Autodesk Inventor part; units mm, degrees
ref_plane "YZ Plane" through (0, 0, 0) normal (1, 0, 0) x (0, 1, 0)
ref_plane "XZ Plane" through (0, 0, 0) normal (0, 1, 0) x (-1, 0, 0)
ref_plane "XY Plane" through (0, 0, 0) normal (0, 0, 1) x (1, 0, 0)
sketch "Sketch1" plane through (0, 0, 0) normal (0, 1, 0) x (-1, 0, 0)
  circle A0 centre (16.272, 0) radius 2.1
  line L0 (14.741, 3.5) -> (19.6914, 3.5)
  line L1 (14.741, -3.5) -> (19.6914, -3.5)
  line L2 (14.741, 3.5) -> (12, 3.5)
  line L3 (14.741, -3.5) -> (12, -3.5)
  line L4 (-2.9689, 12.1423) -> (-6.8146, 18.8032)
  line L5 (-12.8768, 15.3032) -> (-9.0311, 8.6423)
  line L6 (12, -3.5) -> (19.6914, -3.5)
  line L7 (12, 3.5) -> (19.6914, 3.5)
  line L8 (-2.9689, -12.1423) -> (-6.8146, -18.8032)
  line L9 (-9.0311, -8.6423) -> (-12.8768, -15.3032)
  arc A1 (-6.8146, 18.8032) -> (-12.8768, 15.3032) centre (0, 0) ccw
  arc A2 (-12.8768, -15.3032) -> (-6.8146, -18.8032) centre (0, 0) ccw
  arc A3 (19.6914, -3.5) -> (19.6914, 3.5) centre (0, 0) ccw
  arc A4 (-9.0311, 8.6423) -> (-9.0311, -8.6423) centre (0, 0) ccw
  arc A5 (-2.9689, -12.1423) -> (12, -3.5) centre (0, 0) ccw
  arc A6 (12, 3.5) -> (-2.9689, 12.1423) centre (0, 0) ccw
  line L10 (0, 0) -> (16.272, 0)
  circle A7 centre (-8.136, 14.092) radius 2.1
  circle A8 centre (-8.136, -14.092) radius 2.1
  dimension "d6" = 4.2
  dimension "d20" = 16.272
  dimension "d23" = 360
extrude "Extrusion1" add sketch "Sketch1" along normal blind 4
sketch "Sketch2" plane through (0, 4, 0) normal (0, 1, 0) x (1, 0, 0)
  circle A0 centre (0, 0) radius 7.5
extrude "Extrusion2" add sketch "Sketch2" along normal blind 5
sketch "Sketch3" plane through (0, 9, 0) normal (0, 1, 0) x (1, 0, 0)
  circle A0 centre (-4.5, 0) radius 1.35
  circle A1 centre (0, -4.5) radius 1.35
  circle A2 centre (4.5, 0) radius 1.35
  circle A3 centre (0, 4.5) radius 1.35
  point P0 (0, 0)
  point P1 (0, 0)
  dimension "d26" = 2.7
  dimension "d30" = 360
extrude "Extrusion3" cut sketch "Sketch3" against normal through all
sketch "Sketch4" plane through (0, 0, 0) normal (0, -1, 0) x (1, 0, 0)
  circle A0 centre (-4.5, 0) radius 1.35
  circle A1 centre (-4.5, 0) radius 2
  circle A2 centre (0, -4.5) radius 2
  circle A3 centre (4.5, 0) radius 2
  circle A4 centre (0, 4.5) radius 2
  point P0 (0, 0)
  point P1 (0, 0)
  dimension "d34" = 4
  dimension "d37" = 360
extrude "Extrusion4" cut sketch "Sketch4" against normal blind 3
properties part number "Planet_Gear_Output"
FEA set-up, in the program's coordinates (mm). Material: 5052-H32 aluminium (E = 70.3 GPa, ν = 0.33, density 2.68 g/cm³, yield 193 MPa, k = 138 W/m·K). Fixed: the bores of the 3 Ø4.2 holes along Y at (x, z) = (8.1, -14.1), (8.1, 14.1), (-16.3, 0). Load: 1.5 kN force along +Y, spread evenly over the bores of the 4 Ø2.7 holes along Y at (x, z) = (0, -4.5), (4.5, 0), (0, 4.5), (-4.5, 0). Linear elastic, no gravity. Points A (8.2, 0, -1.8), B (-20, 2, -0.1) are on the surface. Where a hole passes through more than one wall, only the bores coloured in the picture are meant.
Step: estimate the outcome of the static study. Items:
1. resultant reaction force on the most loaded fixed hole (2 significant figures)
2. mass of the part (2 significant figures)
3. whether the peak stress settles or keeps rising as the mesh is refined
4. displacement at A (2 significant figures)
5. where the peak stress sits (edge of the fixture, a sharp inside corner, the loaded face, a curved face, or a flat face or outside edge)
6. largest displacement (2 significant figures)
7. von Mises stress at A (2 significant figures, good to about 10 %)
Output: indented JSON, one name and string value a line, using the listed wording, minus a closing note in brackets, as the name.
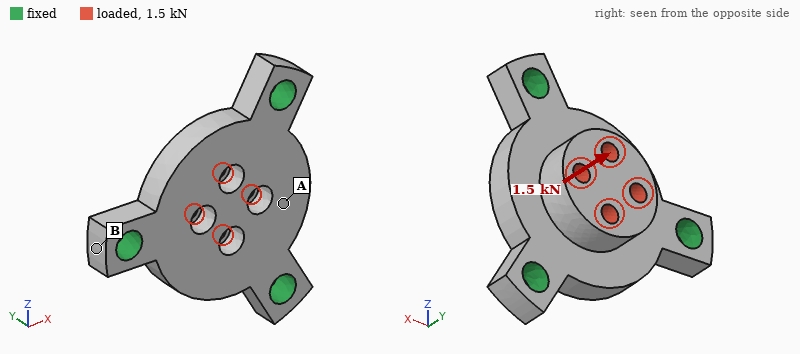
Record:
{
  "resultant reaction force on the most loaded fixed hole": "530 N",
  "mass of the part": "8.1 g",
  "whether the peak stress settles or keeps rising as the mesh is refined": "keeps rising",
  "displacement at A": "14 µm",
  "where the peak stress sits": "edge of the fixture",
  "largest displacement": "17 µm",
  "von Mises stress at A": "35 MPa"
}
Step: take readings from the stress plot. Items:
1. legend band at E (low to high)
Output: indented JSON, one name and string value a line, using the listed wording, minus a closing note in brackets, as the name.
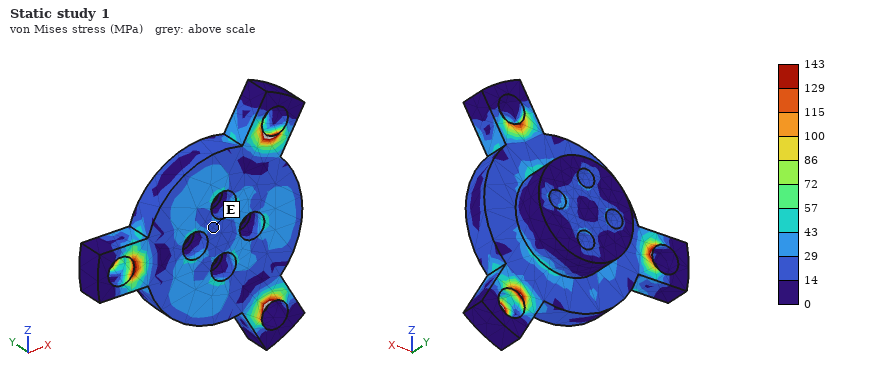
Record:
{
  "legend band at E": "14 to 29 MPa"
}
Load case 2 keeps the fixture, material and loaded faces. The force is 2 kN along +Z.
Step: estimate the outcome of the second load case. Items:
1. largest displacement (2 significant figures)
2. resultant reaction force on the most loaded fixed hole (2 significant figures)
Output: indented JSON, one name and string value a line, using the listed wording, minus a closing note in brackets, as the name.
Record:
{
  "largest displacement": "16 µm",
  "resultant reaction force on the most loaded fixed hole": "940 N"
}
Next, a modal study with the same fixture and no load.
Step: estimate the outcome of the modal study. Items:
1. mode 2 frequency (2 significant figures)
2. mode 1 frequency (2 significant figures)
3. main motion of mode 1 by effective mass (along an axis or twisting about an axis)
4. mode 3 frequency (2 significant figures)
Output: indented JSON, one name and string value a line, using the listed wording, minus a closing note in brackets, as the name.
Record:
{
  "mode 2 frequency": "27 kHz",
  "mode 1 frequency": "21 kHz",
  "main motion of mode 1 by effective mass": "along Y",
  "mode 3 frequency": "27 kHz"
}
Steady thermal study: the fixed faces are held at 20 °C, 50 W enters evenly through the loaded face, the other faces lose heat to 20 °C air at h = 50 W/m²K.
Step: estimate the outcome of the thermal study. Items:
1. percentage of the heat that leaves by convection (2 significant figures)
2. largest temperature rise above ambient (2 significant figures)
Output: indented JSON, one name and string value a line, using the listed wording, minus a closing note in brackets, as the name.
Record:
{
  "percentage of the heat that leaves by convection": "4.3 %",
  "largest temperature rise above ambient": "39 K"
}
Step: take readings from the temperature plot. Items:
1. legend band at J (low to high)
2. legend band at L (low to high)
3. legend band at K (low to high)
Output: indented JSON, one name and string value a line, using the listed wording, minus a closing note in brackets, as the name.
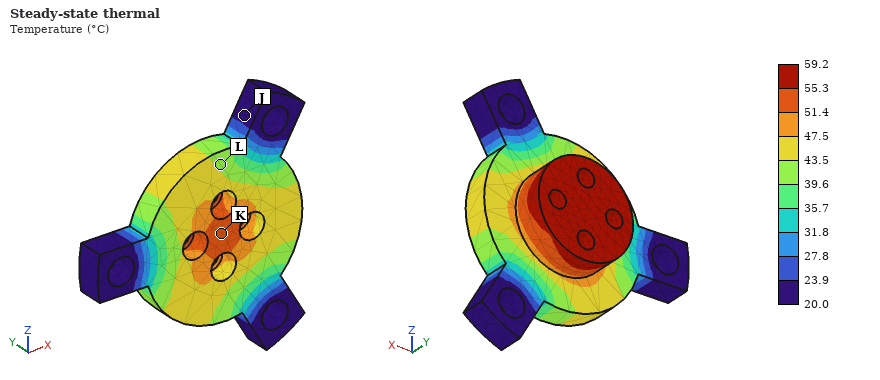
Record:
{
  "legend band at J": "20.0 to 23.9 °C",
  "legend band at L": "39.6 to 43.5 °C",
  "legend band at K": "51.4 to 55.3 °C"
}
